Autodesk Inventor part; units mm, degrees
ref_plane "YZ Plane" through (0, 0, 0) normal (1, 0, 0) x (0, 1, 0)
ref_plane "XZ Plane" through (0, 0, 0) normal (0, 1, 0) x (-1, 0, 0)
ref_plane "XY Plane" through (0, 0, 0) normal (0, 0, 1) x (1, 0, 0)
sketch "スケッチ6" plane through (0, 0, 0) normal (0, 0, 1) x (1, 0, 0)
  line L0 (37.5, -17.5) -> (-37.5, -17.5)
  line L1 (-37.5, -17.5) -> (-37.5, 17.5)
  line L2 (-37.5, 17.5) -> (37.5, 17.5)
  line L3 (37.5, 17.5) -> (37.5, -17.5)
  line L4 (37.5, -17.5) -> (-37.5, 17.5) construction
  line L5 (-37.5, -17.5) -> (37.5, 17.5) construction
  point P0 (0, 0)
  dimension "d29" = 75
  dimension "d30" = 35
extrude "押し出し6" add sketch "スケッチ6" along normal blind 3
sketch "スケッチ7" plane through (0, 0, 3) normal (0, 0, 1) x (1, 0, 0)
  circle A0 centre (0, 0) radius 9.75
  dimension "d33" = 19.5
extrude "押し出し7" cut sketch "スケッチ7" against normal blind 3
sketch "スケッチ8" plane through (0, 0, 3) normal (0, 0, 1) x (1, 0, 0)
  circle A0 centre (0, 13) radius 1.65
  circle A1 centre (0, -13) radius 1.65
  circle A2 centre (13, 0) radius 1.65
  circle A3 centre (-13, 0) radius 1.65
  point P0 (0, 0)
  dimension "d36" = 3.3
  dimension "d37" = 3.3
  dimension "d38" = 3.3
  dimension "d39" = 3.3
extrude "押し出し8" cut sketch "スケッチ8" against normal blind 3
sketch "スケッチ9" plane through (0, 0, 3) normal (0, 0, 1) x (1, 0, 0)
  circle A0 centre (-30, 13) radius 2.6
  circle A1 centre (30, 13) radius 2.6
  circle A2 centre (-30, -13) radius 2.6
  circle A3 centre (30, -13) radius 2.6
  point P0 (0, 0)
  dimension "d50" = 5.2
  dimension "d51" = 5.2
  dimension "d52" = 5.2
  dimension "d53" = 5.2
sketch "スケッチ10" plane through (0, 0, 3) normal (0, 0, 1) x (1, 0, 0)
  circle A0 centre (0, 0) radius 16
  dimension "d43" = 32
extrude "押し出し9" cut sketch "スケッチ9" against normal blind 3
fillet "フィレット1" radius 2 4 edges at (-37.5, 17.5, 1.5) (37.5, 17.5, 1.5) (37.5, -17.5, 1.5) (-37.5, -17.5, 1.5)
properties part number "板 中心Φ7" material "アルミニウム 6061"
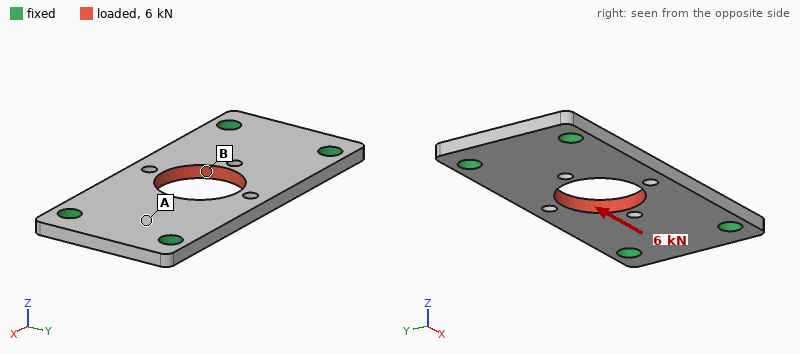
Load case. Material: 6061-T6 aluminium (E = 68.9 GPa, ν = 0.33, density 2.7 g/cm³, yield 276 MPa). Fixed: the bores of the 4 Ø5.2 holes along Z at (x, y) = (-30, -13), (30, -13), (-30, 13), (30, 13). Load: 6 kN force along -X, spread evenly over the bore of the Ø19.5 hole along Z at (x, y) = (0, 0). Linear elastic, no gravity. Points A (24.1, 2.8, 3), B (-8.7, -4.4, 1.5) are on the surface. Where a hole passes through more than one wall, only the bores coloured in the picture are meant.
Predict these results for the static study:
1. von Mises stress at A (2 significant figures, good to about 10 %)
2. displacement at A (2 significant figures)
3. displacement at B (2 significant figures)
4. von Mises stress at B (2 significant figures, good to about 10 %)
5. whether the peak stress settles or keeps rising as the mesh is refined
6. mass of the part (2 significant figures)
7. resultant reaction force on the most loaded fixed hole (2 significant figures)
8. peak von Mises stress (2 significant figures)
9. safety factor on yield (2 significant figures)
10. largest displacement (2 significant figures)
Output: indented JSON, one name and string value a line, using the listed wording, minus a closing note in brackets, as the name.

{
  "von Mises stress at A": "17 MPa",
  "displacement at A": "5.5 µm",
  "displacement at B": "12 µm",
  "von Mises stress at B": "39 MPa",
  "whether the peak stress settles or keeps rising as the mesh is refined": "settles",
  "mass of the part": "18 g",
  "resultant reaction force on the most loaded fixed hole": "1.5 kN",
  "peak von Mises stress": "110 MPa",
  "safety factor on yield": "2.4",
  "largest displacement": "14 µm"
}
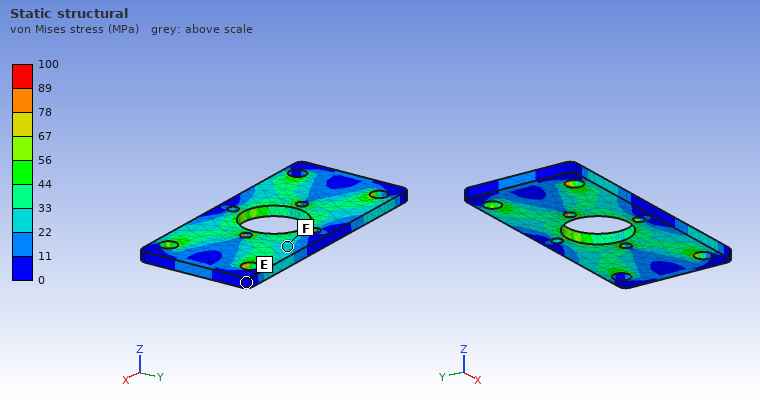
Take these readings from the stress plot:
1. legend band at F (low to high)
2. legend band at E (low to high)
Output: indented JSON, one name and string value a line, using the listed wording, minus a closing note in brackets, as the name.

{
  "legend band at F": "22 to 33 MPa",
  "legend band at E": "0 to 11 MPa"
}
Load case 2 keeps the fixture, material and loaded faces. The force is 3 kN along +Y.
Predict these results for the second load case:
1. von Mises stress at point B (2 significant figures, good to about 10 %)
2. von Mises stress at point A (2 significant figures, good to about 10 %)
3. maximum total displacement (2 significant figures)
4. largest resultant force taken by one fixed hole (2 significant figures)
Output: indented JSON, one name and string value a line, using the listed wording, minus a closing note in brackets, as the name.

{
  "von Mises stress at point B": "40 MPa",
  "von Mises stress at point A": "31 MPa",
  "maximum total displacement": "26 µm",
  "largest resultant force taken by one fixed hole": "1.1 kN"
}
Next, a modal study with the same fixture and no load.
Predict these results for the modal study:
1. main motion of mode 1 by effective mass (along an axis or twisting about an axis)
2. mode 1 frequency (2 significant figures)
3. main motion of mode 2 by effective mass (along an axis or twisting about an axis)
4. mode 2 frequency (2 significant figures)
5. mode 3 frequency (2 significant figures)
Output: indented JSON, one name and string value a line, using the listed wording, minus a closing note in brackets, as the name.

{
  "main motion of mode 1 by effective mass": "along Z",
  "mode 1 frequency": "4900 Hz",
  "main motion of mode 2 by effective mass": "twisting about X",
  "mode 2 frequency": "6700 Hz",
  "mode 3 frequency": "11 kHz"
}
